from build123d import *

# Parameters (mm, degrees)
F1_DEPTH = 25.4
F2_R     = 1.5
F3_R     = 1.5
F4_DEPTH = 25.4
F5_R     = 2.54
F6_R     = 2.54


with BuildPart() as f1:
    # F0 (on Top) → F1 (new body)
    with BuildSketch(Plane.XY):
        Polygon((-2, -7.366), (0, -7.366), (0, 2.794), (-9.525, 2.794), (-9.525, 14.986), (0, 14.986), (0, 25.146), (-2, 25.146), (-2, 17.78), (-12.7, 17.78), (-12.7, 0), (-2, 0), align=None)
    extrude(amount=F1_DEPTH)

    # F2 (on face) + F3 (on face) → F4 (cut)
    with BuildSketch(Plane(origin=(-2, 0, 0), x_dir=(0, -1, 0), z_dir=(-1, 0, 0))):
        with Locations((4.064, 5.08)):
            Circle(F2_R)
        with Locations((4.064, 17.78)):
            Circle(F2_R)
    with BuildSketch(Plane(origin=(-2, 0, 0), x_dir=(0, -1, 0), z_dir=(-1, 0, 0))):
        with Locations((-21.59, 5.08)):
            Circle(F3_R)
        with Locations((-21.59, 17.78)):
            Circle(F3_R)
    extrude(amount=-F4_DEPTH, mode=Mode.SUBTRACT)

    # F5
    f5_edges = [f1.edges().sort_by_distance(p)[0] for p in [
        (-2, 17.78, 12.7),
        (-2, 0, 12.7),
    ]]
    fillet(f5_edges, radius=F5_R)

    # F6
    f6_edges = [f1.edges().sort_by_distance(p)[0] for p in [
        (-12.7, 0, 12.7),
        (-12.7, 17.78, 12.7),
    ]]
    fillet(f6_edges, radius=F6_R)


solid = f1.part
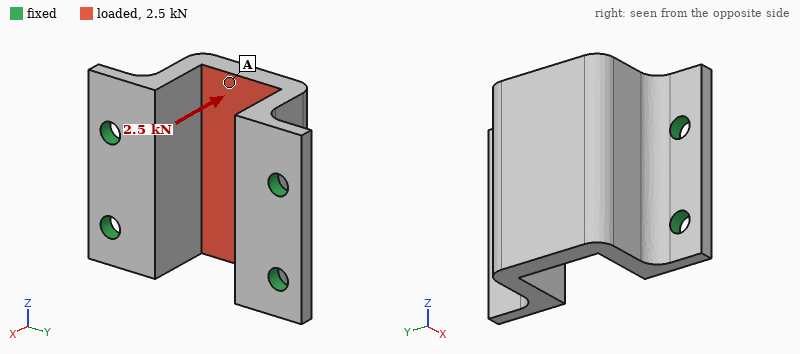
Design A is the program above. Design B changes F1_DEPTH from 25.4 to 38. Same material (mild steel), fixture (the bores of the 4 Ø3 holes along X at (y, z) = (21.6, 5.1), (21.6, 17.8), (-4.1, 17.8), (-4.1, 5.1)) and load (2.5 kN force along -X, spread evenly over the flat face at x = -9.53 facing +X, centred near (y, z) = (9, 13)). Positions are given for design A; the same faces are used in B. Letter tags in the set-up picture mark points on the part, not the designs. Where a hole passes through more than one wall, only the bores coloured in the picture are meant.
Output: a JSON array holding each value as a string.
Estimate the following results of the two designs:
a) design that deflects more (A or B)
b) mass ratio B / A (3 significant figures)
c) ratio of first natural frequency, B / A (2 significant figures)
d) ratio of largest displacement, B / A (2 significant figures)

["B", "1.50", "0.53", "3.3"]
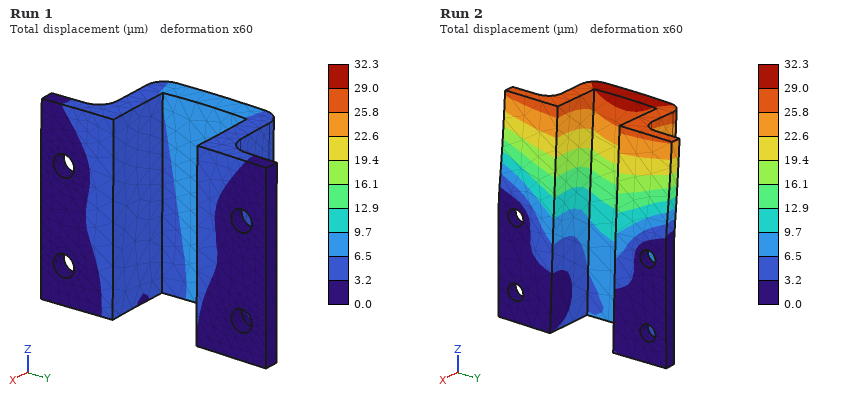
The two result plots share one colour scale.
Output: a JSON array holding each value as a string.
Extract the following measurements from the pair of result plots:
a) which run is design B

["Run 2"]
